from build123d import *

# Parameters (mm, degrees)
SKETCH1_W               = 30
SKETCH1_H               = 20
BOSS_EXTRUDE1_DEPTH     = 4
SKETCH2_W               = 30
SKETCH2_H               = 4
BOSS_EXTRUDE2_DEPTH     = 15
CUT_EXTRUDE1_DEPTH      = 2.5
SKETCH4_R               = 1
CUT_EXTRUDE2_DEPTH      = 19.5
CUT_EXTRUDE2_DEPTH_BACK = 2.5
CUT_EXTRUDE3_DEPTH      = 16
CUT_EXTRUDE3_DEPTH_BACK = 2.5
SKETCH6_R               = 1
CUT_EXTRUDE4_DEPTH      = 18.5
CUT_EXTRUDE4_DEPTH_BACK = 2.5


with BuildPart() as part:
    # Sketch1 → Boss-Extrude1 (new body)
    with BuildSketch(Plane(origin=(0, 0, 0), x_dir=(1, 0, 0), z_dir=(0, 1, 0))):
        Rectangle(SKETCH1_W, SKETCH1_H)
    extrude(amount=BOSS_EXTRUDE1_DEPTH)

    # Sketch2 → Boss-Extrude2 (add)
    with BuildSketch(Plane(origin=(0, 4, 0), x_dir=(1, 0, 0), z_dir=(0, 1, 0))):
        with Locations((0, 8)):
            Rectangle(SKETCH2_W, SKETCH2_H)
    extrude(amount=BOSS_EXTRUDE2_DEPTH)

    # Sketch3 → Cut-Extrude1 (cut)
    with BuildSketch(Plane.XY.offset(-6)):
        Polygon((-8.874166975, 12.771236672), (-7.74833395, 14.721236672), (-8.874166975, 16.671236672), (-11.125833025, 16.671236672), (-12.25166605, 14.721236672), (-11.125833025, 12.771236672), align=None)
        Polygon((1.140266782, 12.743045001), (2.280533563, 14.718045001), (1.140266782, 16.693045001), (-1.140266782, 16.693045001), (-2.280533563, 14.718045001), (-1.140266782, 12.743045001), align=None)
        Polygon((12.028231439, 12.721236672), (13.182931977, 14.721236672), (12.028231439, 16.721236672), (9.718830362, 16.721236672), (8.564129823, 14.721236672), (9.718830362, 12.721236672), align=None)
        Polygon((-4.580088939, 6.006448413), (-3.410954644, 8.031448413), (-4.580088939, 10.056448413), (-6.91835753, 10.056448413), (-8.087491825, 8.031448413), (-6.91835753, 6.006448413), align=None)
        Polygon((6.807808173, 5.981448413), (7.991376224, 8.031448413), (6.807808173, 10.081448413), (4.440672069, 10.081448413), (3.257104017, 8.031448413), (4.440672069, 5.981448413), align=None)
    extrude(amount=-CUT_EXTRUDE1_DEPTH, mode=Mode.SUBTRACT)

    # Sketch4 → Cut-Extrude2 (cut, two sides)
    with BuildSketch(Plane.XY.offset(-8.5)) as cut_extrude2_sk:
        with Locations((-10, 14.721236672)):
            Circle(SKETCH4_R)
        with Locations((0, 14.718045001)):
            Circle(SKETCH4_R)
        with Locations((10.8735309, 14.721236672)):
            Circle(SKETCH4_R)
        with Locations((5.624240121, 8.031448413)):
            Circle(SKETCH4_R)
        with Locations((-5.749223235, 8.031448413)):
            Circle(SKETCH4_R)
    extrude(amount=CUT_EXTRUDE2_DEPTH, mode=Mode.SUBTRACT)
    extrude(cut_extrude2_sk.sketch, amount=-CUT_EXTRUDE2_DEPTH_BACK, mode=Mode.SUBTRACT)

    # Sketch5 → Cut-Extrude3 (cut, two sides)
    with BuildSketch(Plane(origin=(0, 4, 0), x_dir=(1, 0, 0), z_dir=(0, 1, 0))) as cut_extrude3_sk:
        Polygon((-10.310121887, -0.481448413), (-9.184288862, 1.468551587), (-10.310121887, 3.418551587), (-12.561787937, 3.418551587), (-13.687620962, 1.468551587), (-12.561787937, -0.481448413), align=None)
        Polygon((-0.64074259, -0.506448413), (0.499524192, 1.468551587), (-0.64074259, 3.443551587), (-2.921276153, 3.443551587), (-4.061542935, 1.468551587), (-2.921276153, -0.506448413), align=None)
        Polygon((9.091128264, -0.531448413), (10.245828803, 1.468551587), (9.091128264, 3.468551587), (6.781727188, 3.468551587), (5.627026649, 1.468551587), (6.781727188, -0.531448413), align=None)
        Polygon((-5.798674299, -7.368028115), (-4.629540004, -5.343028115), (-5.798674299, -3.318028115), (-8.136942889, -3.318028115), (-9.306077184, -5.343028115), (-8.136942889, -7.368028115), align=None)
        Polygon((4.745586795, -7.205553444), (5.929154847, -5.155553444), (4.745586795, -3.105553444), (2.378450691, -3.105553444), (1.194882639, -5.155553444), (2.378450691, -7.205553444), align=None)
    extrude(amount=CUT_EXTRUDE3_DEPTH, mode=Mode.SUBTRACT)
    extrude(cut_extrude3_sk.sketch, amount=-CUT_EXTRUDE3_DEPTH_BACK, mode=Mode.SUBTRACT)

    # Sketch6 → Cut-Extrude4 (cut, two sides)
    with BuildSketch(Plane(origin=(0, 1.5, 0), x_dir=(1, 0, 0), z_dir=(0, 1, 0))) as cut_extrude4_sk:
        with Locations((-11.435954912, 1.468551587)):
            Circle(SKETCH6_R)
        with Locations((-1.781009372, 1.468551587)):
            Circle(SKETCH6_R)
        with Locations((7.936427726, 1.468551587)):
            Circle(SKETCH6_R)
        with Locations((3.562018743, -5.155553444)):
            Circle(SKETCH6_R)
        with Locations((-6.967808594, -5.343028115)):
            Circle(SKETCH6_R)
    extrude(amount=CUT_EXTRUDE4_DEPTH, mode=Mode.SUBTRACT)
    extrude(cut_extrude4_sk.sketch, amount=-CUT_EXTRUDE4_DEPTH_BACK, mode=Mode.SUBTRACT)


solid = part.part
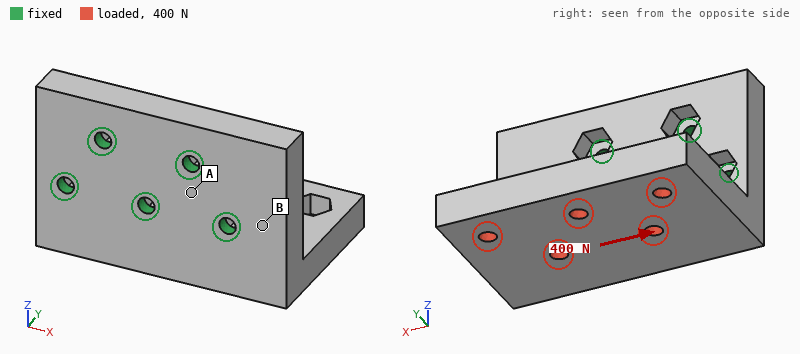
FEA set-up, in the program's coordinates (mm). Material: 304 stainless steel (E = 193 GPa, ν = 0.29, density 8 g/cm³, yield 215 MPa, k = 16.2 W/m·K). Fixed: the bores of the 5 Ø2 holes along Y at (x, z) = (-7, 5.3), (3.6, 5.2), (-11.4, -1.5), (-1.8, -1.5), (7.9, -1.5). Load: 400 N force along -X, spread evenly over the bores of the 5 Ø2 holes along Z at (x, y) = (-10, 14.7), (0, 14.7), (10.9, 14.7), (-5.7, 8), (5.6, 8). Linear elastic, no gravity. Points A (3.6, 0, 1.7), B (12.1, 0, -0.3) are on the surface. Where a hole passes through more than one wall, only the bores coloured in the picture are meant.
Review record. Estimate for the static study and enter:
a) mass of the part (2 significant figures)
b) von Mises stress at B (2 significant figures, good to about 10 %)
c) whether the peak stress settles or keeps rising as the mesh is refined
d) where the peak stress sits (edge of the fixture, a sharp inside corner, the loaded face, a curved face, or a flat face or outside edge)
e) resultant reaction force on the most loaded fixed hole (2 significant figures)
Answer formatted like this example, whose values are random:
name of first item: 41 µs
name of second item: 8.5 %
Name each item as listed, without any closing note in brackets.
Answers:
mass of the part: 30 g
von Mises stress at B: 15 MPa
whether the peak stress settles or keeps rising as the mesh is refined: keeps rising
where the peak stress sits: edge of the fixture
resultant reaction force on the most loaded fixed hole: 310 N
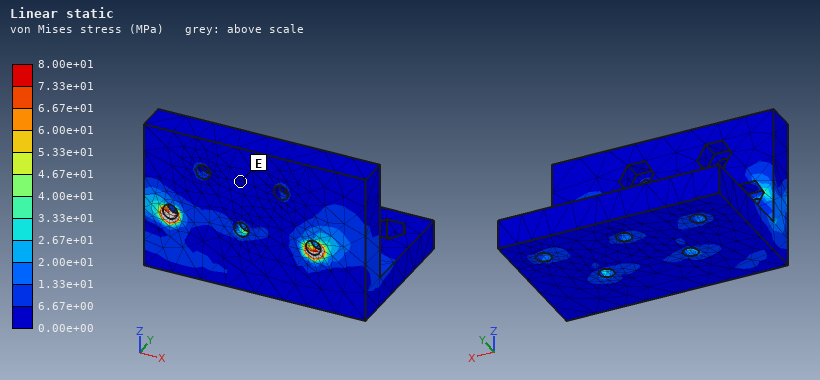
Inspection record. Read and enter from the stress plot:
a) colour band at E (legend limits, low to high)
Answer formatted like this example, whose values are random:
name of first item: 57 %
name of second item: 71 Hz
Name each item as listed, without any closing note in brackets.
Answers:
colour band at E: 0.00e+00 to 6.67e+00 MPa
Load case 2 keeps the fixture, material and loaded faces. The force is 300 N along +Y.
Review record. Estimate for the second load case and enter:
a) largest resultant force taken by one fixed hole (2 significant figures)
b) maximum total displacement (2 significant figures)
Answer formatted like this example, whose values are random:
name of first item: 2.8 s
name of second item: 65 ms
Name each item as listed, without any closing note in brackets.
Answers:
largest resultant force taken by one fixed hole: 210 N
maximum total displacement: 13 µm
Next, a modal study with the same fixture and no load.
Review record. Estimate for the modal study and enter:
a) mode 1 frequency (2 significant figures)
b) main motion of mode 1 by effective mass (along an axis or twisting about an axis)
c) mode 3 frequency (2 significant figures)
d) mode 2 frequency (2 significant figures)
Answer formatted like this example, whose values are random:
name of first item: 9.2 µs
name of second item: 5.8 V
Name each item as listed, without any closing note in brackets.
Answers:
mode 1 frequency: 5600 Hz
main motion of mode 1 by effective mass: along Z
mode 3 frequency: 16 kHz
mode 2 frequency: 10 kHz
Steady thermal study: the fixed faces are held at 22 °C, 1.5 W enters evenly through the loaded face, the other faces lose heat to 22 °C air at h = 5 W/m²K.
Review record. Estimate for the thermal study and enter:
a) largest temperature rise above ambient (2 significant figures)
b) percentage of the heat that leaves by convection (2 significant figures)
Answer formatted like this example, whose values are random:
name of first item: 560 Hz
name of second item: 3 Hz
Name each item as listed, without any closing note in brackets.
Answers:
largest temperature rise above ambient: 17 K
percentage of the heat that leaves by convection: 6.8 %
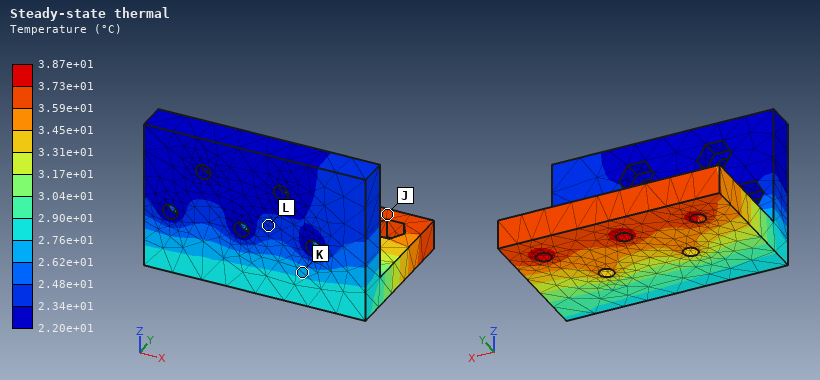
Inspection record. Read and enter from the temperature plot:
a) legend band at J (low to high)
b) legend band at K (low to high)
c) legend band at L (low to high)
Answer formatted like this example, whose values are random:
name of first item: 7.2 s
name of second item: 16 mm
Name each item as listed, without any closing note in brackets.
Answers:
legend band at J: 3.59e+01 to 3.73e+01 °C
legend band at K: 2.62e+01 to 2.76e+01 °C
legend band at L: 2.34e+01 to 2.48e+01 °C
